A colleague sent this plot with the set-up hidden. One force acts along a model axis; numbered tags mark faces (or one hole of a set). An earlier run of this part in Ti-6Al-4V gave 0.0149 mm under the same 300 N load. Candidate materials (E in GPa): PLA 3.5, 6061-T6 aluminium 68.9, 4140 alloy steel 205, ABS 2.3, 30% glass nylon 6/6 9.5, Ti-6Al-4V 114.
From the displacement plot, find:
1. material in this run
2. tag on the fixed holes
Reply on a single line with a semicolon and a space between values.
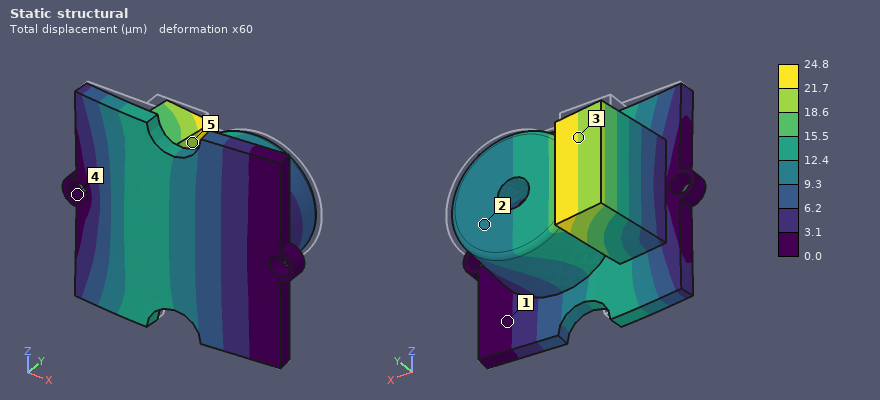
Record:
6061-T6 aluminium; 4
